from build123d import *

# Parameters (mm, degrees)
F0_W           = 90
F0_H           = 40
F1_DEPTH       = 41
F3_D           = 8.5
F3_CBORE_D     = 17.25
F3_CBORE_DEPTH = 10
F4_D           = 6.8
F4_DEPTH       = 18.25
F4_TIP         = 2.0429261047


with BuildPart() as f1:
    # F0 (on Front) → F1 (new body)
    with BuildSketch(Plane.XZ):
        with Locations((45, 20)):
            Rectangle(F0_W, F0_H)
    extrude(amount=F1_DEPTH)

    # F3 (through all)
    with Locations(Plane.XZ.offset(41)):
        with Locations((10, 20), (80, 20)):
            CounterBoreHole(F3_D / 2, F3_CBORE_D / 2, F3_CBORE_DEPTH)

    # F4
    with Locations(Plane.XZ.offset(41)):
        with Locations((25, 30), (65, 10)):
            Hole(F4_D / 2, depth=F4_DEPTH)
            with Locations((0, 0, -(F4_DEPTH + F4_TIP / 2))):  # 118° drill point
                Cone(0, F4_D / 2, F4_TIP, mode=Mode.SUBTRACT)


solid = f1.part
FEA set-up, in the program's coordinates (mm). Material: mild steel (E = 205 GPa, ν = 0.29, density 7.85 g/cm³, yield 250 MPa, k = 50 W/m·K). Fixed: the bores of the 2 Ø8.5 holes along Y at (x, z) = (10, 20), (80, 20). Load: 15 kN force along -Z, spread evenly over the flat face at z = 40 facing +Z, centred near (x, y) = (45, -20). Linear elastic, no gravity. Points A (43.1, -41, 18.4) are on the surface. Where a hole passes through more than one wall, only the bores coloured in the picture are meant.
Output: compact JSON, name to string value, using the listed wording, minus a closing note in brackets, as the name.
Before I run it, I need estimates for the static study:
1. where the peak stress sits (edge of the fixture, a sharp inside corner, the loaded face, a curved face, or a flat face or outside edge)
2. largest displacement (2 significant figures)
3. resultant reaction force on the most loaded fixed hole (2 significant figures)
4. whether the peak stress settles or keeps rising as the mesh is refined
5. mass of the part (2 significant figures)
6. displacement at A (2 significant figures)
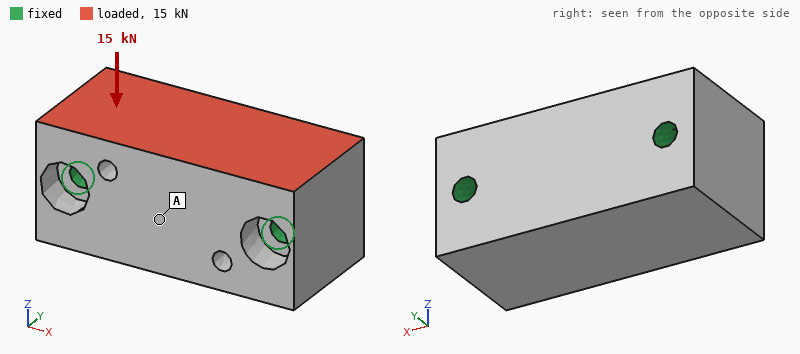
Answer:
{"where the peak stress sits": "edge of the fixture", "largest displacement": "3.0 µm", "resultant reaction force on the most loaded fixed hole": "7.5 kN", "whether the peak stress settles or keeps rising as the mesh is refined": "keeps rising", "mass of the part": "1.1 kg", "displacement at A": "2.5 µm"}
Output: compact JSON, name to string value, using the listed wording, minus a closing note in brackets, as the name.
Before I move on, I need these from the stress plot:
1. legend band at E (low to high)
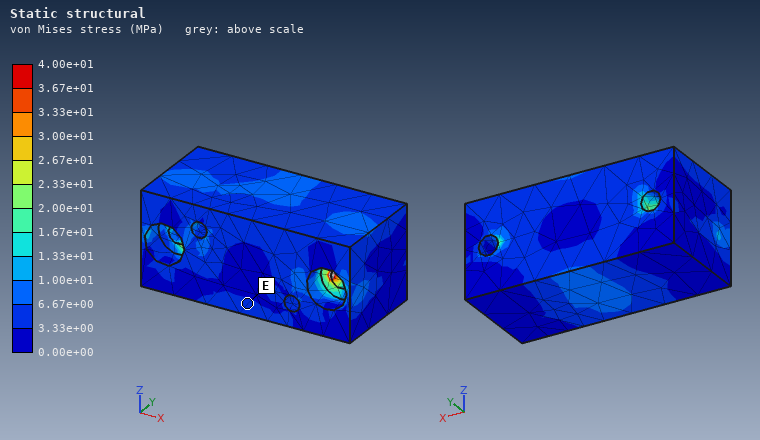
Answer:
{"legend band at E": "3.33e+00 to 6.67e+00 MPa"}
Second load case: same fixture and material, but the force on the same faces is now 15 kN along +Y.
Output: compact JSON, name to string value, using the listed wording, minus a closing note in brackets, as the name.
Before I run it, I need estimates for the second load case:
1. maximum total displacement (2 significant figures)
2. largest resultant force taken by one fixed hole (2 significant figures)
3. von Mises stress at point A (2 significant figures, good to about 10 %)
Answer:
{"maximum total displacement": "6.7 µm", "largest resultant force taken by one fixed hole": "7.6 kN", "von Mises stress at point A": "7.0 MPa"}
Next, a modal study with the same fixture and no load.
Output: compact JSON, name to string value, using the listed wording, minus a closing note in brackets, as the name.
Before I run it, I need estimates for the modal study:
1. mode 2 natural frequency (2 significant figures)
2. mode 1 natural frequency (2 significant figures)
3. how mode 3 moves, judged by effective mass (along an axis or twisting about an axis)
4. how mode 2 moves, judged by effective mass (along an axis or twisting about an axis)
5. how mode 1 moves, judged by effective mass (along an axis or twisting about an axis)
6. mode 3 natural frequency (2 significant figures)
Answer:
{"mode 2 natural frequency": "15 kHz", "mode 1 natural frequency": "13 kHz", "how mode 3 moves, judged by effective mass": "along Z", "how mode 2 moves, judged by effective mass": "along Y", "how mode 1 moves, judged by effective mass": "along Z", "mode 3 natural frequency": "16 kHz"}
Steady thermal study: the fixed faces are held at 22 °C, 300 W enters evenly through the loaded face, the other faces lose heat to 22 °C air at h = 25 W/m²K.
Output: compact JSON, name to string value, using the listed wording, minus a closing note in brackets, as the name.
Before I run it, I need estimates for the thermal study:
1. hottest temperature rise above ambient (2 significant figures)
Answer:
{"hottest temperature rise above ambient": "61 K"}
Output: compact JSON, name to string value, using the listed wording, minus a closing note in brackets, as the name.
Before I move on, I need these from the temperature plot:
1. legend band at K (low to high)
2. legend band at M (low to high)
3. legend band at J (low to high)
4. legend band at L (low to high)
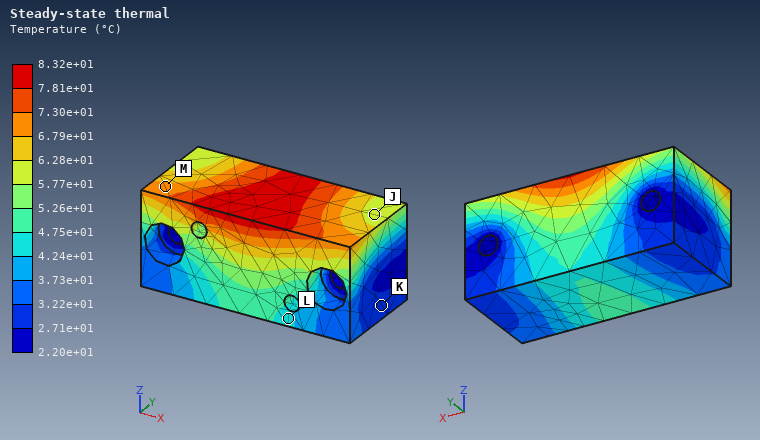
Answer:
{"legend band at K": "2.71e+01 to 3.22e+01 °C", "legend band at M": "6.79e+01 to 7.30e+01 °C", "legend band at J": "5.77e+01 to 6.28e+01 °C", "legend band at L": "4.24e+01 to 4.75e+01 °C"}
